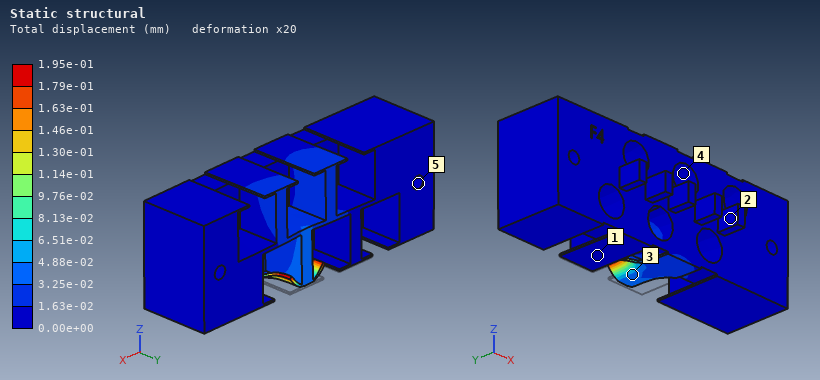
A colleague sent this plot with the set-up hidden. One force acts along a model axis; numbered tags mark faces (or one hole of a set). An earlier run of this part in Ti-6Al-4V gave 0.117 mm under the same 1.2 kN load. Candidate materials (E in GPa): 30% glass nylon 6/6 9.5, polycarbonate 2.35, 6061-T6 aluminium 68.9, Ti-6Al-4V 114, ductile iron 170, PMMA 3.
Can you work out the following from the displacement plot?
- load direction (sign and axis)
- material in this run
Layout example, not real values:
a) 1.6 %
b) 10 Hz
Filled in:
a) +Z
b) 6061-T6 aluminium
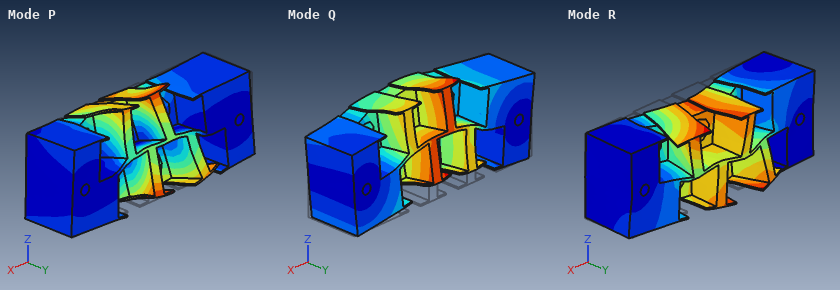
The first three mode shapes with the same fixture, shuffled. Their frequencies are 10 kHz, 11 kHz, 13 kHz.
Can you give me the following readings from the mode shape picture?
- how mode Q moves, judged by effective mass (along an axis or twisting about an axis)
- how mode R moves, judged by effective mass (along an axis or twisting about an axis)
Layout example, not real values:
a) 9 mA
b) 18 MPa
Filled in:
a) along Z
b) along Y
